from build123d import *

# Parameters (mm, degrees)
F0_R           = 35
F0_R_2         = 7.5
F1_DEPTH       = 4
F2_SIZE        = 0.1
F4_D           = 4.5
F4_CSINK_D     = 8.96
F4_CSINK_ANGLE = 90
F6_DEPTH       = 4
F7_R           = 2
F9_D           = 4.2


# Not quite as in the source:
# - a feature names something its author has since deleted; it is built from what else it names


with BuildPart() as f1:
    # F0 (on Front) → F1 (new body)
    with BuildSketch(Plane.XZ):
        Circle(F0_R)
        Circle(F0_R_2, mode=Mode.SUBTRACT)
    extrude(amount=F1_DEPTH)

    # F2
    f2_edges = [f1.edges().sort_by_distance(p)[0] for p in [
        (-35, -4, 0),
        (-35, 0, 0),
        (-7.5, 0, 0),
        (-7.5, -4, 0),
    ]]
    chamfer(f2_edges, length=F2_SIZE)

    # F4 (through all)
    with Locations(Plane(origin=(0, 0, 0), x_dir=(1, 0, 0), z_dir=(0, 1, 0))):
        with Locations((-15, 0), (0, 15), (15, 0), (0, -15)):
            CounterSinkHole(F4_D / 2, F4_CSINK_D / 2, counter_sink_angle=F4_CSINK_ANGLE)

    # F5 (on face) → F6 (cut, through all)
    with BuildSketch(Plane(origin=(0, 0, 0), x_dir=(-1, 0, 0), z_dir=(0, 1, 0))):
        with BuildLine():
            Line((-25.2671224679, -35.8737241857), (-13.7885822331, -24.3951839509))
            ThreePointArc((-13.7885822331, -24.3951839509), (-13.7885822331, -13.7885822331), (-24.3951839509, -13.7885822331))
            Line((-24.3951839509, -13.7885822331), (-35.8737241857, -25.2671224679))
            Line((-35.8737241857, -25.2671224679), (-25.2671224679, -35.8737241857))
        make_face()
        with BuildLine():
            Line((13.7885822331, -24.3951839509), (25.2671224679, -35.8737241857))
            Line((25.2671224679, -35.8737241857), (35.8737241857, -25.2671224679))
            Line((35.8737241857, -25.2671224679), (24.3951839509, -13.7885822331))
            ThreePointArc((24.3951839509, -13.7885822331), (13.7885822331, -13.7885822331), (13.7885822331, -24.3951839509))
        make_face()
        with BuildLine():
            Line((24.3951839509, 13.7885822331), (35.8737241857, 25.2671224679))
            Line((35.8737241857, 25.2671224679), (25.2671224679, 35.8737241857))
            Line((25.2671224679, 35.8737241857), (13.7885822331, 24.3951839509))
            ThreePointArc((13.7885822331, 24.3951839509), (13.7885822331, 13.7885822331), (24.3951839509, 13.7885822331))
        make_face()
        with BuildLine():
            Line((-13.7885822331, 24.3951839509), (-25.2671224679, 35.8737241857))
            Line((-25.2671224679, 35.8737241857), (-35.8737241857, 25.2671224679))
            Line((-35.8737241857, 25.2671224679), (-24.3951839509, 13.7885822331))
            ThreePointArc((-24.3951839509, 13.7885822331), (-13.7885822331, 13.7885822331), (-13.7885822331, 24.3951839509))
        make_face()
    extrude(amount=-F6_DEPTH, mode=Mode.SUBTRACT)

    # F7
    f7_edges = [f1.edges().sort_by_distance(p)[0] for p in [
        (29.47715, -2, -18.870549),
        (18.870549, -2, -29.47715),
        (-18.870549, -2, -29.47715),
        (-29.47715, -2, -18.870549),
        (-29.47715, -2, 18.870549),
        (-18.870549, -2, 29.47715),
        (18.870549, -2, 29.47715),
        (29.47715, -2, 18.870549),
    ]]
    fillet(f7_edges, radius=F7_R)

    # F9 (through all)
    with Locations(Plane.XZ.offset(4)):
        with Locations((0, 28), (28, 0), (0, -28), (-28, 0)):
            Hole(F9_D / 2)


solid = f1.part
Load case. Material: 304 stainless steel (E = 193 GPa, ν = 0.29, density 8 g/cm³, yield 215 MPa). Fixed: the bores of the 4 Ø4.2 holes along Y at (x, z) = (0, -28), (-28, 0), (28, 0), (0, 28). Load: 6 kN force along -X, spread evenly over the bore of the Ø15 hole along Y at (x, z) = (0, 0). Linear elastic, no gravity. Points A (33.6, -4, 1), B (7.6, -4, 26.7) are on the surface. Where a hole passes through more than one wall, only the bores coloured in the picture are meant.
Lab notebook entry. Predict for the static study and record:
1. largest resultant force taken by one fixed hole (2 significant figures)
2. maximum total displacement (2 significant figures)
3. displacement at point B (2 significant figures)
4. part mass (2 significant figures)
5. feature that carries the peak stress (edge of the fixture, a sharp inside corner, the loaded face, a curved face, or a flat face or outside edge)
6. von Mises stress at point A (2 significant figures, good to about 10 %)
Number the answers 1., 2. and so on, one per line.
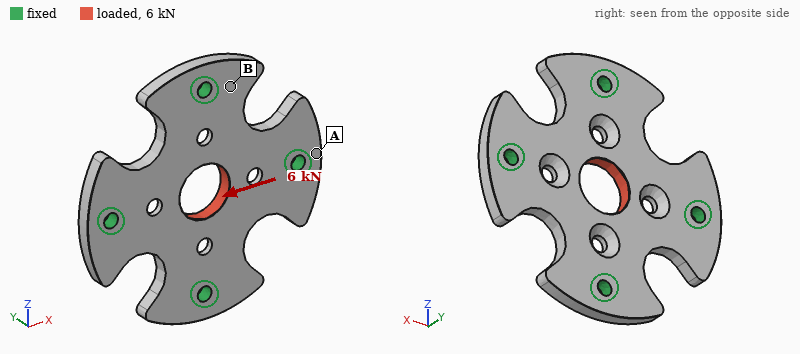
1. 2.5 kN
2. 6.0 µm
3. 1.2 µm
4. 86 g
5. a curved face
6. 28 MPa
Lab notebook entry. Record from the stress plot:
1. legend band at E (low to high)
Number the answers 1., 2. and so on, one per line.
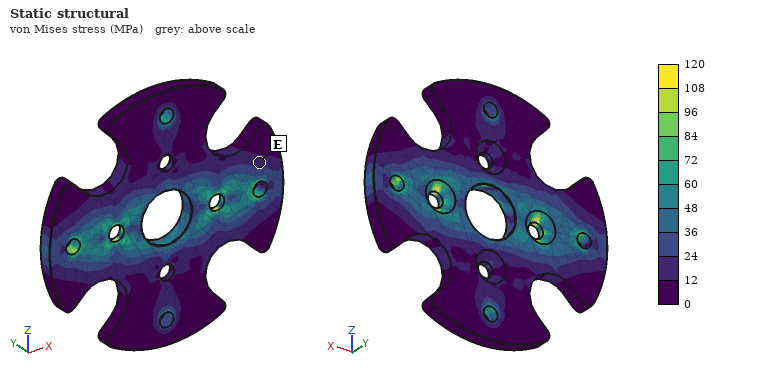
1. 12 to 24 MPa
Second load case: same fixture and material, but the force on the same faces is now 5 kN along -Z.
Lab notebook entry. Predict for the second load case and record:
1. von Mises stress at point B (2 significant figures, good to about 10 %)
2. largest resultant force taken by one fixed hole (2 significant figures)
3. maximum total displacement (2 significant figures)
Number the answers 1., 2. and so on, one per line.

1. 16 MPa
2. 2.1 kN
3. 5.0 µm
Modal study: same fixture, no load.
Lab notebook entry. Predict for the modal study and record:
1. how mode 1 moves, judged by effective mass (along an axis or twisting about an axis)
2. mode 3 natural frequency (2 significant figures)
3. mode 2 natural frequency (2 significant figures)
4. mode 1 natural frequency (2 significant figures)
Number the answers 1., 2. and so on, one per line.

1. along Y
2. 14 kHz
3. 14 kHz
4. 9600 Hz
